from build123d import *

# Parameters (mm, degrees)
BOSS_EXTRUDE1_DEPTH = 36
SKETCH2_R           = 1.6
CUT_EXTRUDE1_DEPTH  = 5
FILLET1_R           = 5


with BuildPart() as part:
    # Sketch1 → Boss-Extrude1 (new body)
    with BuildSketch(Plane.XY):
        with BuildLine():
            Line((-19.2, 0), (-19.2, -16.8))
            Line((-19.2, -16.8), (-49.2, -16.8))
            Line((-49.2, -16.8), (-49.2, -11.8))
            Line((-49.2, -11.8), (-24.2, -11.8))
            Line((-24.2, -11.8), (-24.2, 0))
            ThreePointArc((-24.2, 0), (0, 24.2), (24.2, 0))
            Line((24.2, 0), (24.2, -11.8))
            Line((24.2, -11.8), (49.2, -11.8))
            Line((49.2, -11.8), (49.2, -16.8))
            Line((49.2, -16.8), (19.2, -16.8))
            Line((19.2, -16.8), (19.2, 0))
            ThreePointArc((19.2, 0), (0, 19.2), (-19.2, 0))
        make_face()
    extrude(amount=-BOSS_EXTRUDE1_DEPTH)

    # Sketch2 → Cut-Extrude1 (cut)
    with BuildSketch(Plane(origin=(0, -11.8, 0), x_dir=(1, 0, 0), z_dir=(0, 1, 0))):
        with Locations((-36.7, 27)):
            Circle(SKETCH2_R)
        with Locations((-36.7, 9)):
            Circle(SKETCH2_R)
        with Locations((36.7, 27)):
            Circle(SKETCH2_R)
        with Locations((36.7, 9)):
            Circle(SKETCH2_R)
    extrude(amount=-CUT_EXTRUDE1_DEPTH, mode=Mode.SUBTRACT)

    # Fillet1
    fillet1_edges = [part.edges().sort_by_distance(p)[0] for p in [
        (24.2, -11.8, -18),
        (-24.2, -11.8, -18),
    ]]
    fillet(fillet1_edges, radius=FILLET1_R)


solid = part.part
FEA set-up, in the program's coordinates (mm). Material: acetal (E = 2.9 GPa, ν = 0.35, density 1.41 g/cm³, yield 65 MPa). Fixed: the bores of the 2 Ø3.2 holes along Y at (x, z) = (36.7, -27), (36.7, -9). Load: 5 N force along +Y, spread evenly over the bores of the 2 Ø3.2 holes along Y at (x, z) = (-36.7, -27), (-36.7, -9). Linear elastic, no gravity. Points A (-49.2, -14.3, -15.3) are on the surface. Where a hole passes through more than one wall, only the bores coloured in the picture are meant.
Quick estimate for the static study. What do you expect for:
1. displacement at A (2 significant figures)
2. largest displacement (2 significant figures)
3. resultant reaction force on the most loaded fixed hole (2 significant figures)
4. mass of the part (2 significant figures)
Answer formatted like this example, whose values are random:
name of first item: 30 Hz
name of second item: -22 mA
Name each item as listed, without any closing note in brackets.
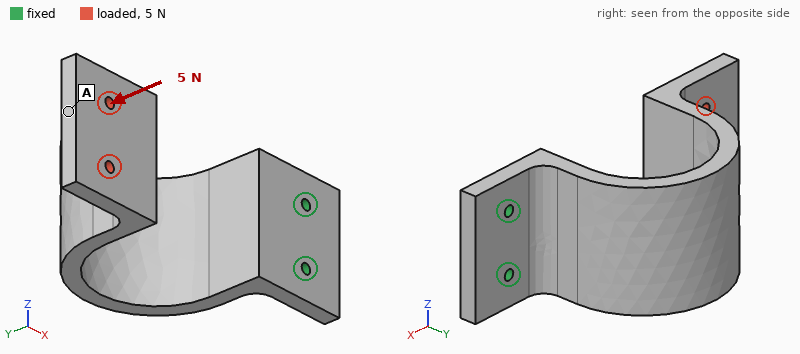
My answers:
displacement at A: 1.2 mm
largest displacement: 1.2 mm
resultant reaction force on the most loaded fixed hole: 3.1 N
mass of the part: 39 g
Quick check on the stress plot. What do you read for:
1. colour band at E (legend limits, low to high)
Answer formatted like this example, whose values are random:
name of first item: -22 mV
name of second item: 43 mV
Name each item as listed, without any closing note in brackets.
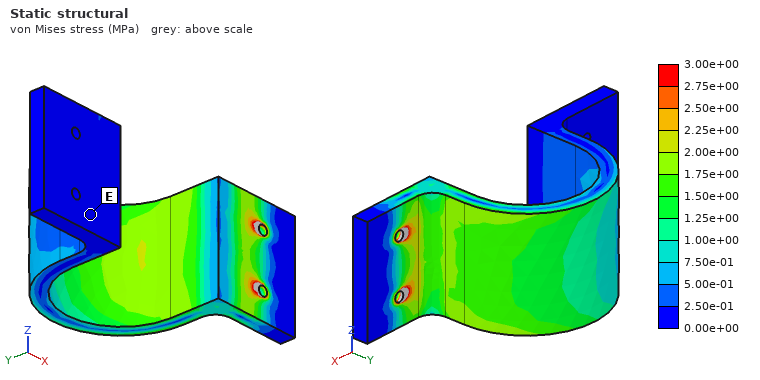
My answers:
colour band at E: 0.00e+00 to 2.50e-01 MPa
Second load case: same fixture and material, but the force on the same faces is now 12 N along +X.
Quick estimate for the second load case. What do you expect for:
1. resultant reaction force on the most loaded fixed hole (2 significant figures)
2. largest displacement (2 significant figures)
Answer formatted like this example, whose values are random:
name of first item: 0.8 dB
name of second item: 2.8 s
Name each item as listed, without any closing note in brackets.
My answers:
resultant reaction force on the most loaded fixed hole: 6.0 N
largest displacement: 1.3 mm
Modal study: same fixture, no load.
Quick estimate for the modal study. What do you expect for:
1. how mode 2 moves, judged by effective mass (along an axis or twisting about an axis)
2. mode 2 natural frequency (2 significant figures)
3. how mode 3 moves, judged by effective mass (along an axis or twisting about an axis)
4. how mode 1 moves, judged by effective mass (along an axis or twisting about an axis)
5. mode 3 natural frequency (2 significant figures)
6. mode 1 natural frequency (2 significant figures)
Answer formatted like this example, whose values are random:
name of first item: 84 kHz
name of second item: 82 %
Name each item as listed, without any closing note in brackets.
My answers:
how mode 2 moves, judged by effective mass: along Z
mode 2 natural frequency: 160 Hz
how mode 3 moves, judged by effective mass: along X
how mode 1 moves, judged by effective mass: along Y
mode 3 natural frequency: 250 Hz
mode 1 natural frequency: 100 Hz
